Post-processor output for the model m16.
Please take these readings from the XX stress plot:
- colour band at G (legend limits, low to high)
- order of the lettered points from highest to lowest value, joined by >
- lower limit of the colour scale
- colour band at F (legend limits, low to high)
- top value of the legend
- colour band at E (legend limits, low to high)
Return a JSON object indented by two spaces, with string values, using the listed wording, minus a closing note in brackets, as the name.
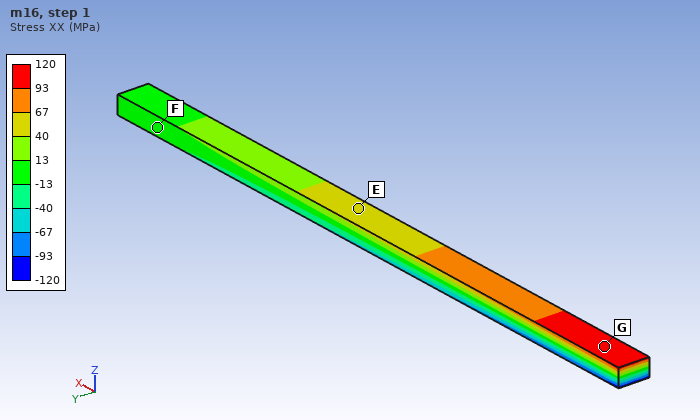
{
  "colour band at G": "93 to 120 MPa",
  "order of the lettered points from highest to lowest value, joined by >": "G > E > F",
  "lower limit of the colour scale": "-120 MPa",
  "colour band at F": "-13 to 13 MPa",
  "top value of the legend": "120 MPa",
  "colour band at E": "40 to 67 MPa"
}
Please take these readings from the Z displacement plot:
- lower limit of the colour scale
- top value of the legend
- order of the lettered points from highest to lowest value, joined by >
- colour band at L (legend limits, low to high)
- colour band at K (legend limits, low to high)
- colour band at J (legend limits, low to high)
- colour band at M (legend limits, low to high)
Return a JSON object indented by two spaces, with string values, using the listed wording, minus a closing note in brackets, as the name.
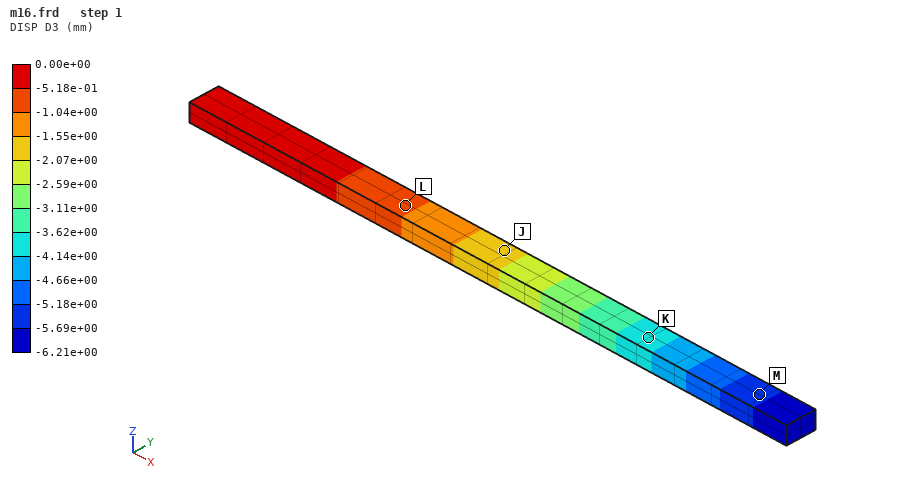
{
  "lower limit of the colour scale": "-6.21e+00 mm",
  "top value of the legend": "0.00e+00 mm",
  "order of the lettered points from highest to lowest value, joined by >": "L > J > K > M",
  "colour band at L": "-1.04e+00 to -5.18e-01 mm",
  "colour band at K": "-4.14e+00 to -3.62e+00 mm",
  "colour band at J": "-2.07e+00 to -1.55e+00 mm",
  "colour band at M": "-5.69e+00 to -5.18e+00 mm"
}
